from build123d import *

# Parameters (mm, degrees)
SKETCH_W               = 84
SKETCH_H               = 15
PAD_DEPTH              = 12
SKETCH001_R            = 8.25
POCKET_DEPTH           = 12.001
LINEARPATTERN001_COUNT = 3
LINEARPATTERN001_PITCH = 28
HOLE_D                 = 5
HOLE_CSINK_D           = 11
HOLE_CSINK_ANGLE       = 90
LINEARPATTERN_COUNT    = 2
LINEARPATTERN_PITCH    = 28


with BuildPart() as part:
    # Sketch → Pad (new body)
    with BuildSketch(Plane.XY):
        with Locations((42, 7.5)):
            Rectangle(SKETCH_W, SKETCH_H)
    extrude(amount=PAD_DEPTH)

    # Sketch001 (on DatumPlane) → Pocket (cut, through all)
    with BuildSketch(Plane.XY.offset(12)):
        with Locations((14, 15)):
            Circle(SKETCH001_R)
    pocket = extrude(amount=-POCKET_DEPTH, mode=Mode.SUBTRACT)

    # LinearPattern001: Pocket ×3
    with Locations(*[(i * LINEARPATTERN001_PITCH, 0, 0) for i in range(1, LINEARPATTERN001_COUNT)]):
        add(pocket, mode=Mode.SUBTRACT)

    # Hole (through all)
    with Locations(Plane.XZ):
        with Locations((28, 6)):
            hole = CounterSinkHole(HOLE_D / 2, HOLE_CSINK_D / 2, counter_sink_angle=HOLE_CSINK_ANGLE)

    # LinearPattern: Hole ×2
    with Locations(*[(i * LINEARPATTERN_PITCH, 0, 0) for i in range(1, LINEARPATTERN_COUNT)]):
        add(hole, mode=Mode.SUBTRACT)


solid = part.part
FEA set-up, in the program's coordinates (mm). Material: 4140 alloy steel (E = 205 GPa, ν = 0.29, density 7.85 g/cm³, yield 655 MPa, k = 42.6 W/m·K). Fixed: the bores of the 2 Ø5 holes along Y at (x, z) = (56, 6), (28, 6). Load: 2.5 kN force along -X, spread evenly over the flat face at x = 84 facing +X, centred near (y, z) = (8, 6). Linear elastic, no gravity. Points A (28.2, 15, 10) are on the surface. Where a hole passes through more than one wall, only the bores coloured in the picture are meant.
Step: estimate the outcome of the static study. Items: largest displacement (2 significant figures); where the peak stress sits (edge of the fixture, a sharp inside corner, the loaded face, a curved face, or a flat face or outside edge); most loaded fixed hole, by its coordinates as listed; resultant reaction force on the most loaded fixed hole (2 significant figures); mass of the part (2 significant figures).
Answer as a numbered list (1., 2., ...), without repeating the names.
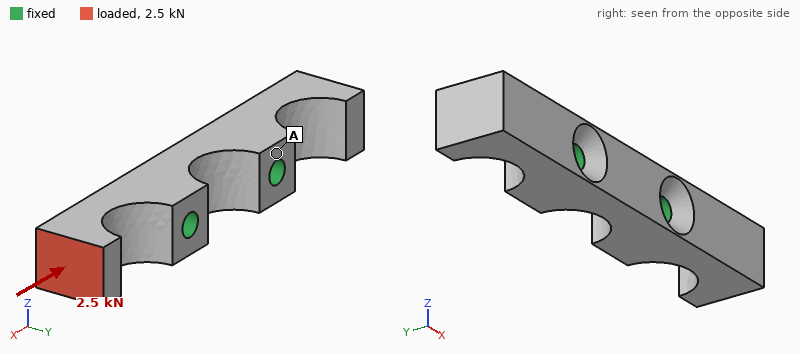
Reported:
1. 36 µm
2. a curved face
3. (56, 6)
4. 2.4 kN
5. 82 g
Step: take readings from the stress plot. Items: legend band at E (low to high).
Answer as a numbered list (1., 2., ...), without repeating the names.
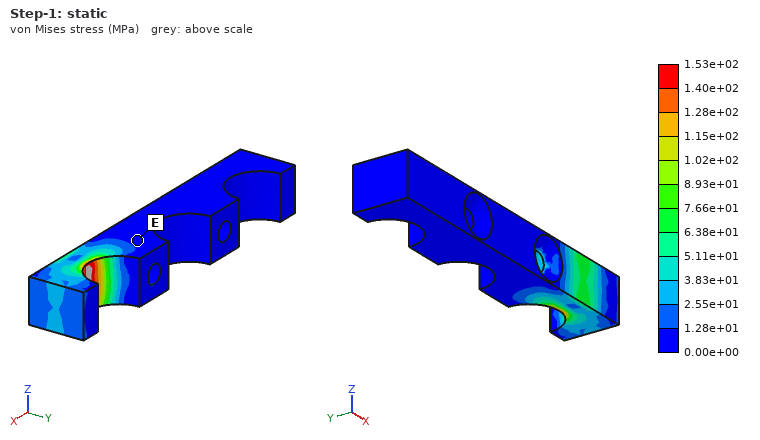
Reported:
1. 0.00e+00 to 1.28e+01 MPa
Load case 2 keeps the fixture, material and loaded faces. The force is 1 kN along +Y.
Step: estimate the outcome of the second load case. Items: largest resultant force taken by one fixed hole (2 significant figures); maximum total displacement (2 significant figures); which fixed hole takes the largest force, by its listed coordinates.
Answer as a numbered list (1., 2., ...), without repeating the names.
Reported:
1. 1.1 kN
2. 68 µm
3. (56, 6)
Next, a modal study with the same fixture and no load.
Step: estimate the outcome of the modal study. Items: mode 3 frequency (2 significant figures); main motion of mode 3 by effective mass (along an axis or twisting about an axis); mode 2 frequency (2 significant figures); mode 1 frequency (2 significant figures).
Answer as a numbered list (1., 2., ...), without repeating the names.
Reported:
1. 8300 Hz
2. along Z
3. 7300 Hz
4. 7300 Hz
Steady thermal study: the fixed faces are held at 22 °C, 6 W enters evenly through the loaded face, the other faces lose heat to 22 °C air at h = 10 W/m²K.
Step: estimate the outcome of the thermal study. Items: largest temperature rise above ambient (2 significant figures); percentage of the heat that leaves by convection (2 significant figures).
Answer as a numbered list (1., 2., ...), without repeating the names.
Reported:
1. 37 K
2. 4.2 %
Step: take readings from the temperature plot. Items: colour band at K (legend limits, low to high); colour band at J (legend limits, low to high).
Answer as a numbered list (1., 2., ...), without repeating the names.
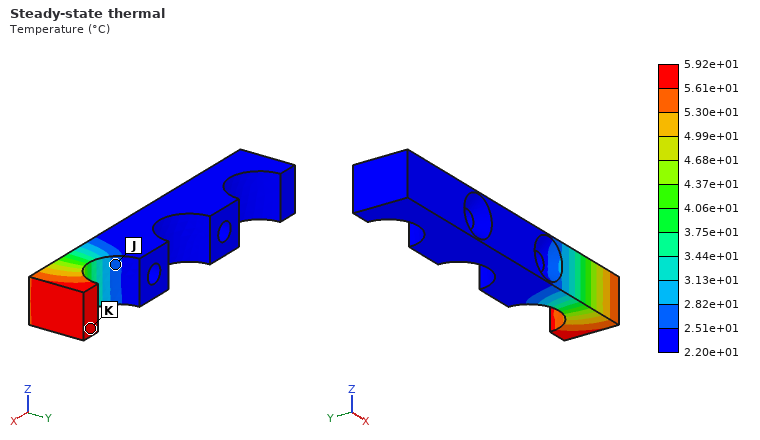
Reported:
1. 5.61e+01 to 5.92e+01 °C
2. 2.51e+01 to 2.82e+01 °C
